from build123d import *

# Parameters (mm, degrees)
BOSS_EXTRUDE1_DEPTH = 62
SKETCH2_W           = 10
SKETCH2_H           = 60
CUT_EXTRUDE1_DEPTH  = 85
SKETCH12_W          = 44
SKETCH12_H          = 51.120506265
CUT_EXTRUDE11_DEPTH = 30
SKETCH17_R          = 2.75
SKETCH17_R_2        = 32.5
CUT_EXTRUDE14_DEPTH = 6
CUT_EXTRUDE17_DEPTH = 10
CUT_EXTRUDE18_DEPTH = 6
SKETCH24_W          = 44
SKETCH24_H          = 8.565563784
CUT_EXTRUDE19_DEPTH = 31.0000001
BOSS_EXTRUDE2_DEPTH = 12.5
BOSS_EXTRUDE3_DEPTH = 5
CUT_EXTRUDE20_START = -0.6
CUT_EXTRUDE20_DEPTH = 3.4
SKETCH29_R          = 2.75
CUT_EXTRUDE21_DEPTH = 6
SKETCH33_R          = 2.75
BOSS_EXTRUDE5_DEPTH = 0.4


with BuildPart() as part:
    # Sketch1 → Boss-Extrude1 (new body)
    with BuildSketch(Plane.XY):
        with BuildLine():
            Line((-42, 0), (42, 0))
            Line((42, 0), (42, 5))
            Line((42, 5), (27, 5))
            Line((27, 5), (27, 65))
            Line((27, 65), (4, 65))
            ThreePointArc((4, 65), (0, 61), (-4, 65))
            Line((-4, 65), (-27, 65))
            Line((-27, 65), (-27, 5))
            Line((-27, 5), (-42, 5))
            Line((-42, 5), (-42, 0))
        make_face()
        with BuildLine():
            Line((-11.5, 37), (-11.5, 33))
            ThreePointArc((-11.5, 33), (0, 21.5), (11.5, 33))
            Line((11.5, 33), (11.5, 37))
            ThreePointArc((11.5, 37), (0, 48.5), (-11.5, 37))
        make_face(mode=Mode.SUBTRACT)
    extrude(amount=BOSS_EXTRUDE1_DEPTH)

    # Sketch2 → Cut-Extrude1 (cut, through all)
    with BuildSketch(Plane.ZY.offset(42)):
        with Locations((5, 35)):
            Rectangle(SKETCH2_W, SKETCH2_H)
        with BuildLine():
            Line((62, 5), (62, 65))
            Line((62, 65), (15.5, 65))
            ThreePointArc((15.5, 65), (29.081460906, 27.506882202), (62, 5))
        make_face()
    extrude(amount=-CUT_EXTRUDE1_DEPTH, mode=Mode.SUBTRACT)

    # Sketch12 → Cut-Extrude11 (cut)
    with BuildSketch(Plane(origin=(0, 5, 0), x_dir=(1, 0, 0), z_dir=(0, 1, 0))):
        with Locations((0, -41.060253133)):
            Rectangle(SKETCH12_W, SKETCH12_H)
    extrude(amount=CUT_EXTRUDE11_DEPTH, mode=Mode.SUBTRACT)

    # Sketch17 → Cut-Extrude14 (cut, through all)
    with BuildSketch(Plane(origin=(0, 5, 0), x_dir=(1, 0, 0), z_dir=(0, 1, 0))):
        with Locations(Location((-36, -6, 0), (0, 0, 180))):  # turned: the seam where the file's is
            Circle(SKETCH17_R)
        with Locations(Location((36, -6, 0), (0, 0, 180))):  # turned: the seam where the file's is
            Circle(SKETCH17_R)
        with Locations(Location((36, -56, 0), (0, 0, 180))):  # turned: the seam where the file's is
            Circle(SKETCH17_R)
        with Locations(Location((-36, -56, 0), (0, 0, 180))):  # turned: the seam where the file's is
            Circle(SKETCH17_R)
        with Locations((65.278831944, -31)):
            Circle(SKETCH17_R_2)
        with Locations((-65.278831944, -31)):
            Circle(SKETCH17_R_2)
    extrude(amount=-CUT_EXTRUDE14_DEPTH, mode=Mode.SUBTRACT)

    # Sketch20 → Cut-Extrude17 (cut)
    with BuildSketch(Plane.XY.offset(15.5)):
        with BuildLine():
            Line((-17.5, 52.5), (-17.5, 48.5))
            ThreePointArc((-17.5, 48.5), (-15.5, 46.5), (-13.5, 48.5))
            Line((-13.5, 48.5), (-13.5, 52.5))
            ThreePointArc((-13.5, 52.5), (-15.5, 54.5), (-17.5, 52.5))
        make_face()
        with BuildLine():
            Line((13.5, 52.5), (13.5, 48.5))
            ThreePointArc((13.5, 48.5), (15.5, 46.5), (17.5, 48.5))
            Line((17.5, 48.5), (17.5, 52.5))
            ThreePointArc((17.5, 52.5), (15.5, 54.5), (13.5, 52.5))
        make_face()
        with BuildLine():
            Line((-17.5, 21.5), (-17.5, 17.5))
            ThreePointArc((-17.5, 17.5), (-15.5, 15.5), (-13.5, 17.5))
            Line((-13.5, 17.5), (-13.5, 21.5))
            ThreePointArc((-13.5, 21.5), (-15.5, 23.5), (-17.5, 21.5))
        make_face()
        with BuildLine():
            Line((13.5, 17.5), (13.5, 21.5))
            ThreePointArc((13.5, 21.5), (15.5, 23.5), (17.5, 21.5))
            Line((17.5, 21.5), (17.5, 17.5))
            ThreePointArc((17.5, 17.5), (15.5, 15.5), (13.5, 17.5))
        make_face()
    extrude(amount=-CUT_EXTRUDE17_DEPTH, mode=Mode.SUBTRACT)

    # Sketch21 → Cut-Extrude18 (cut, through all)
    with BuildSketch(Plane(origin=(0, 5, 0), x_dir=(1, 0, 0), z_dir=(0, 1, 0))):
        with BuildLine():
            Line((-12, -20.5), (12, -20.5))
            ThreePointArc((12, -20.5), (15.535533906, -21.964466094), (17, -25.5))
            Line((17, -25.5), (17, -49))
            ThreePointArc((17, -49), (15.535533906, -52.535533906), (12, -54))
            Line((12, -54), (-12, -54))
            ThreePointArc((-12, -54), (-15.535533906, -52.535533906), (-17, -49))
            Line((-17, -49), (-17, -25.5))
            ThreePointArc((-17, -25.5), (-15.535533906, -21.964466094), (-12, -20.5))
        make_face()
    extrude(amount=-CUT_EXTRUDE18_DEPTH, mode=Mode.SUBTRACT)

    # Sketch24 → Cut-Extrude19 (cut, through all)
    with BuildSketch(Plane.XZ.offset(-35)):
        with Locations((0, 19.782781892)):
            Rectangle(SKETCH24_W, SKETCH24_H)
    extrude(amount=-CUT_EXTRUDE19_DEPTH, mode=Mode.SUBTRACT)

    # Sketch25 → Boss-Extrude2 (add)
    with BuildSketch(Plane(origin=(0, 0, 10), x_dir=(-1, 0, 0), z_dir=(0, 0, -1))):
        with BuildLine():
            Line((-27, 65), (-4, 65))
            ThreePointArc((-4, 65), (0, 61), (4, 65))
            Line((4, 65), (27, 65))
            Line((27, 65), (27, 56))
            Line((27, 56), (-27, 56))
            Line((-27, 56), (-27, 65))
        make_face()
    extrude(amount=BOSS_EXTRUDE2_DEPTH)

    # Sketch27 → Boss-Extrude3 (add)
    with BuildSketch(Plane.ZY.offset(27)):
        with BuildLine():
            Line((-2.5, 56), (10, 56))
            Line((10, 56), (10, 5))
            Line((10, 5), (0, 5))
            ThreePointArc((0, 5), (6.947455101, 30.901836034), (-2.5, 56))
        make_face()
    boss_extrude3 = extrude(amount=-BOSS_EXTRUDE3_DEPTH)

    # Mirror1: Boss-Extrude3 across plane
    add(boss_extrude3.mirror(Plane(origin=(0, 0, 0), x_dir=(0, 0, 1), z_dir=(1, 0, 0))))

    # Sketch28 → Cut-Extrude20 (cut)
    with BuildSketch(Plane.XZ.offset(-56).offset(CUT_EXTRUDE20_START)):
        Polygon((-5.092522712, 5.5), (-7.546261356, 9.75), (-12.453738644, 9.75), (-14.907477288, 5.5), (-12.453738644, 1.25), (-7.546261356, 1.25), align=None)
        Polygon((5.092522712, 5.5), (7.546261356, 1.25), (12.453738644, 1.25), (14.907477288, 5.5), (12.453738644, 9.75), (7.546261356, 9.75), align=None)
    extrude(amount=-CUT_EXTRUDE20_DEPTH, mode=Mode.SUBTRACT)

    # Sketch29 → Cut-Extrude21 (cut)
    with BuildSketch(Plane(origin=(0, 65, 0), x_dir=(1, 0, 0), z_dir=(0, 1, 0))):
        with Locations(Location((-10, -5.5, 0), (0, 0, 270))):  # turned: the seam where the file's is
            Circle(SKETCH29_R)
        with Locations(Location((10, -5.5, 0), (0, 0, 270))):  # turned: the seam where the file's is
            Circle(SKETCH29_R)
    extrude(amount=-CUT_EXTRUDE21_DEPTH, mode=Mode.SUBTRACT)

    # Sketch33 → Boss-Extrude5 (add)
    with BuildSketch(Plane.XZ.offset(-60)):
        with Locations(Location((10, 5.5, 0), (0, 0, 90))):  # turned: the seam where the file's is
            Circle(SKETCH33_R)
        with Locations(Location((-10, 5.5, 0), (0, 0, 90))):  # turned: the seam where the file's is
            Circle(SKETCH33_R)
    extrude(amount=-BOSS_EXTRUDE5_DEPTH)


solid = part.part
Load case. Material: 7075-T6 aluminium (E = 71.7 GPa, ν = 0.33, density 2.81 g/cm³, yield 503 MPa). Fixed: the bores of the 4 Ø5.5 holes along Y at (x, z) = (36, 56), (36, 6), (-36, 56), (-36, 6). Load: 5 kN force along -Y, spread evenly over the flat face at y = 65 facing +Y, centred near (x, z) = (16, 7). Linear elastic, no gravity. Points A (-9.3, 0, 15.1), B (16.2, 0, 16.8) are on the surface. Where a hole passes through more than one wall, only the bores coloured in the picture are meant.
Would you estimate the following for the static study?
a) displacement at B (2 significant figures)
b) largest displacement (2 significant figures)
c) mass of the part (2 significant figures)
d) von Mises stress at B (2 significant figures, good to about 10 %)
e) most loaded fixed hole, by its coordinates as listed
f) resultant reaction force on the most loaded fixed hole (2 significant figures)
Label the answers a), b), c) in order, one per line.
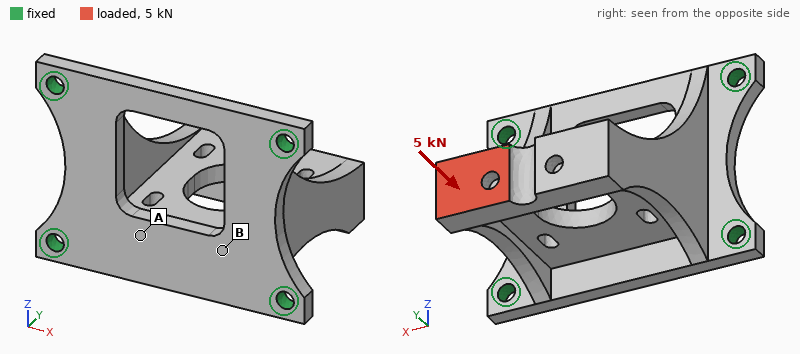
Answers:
a) 0.047 mm
b) 0.29 mm
c) 130 g
d) 29 MPa
e) (36, 6)
f) 3.8 kN
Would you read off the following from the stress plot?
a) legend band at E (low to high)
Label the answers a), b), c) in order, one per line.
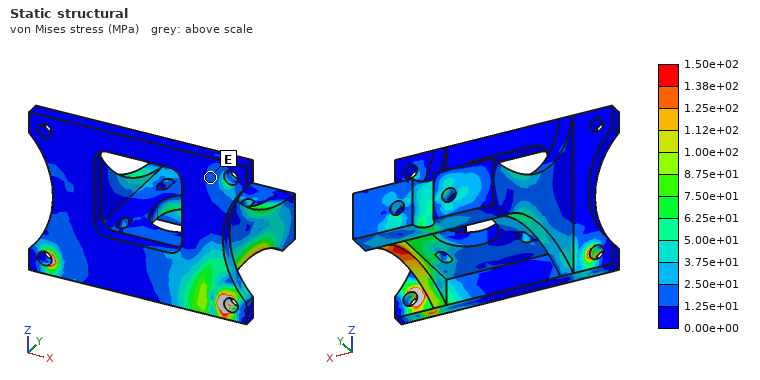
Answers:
a) 1.25e+01 to 2.50e+01 MPa
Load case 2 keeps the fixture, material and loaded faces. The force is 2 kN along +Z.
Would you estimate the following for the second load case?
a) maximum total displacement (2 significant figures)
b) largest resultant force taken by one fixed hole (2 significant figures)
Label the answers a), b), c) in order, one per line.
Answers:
a) 0.45 mm
b) 2.1 kN
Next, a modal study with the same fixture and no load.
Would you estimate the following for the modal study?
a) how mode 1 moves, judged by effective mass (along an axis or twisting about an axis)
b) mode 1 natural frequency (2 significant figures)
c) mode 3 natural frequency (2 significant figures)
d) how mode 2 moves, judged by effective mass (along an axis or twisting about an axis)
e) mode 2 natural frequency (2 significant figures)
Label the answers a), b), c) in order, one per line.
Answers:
a) along Z
b) 2600 Hz
c) 4400 Hz
d) along X
e) 3900 Hz
